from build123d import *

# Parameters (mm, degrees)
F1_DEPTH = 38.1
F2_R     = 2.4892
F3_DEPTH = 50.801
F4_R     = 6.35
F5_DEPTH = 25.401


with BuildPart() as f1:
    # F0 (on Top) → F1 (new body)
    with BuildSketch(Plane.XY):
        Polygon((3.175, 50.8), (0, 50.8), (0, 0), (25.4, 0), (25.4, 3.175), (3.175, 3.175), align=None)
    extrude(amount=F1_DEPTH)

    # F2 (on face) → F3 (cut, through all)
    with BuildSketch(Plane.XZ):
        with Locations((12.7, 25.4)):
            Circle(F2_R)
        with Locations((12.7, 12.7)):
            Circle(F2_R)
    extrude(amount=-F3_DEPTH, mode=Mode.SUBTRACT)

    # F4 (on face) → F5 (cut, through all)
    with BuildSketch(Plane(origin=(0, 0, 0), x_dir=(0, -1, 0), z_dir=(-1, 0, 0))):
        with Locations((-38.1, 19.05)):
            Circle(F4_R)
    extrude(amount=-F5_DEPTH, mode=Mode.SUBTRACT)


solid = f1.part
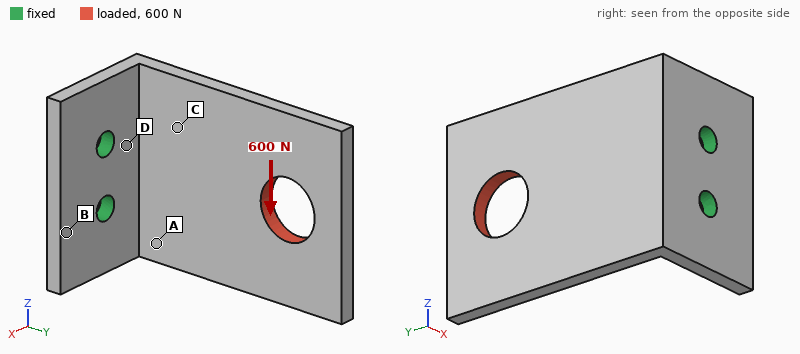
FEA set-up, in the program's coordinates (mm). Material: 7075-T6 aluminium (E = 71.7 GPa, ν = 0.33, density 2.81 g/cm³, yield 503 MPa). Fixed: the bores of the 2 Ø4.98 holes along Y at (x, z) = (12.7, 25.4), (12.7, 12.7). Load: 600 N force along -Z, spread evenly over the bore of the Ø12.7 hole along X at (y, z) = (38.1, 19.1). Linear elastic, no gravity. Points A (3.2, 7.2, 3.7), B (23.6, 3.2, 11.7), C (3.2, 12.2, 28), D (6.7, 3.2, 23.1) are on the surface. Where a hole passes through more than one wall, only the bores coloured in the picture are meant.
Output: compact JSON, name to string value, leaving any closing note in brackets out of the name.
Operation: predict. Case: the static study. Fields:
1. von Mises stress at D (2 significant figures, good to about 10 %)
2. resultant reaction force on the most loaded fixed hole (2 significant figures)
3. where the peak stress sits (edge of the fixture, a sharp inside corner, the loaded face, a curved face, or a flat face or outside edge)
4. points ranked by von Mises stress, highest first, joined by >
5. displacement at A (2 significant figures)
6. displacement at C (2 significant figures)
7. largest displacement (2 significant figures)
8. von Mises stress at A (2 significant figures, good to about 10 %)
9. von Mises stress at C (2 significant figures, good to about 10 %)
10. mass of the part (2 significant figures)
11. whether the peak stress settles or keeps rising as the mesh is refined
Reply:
{"von Mises stress at D": "130 MPa", "resultant reaction force on the most loaded fixed hole": "1.2 kN", "where the peak stress sits": "edge of the fixture", "points ranked by von Mises stress, highest first, joined by >": "D > A > C > B", "displacement at A": "0.12 mm", "displacement at C": "0.11 mm", "largest displacement": "0.42 mm", "von Mises stress at A": "83 MPa", "von Mises stress at C": "51 MPa", "mass of the part": "23 g", "whether the peak stress settles or keeps rising as the mesh is refined": "keeps rising"}
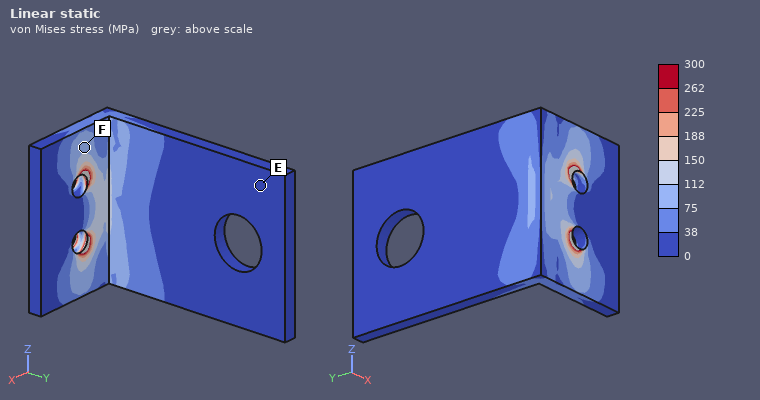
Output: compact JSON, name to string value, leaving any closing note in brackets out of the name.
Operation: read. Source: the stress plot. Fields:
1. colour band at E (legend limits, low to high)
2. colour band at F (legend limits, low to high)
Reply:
{"colour band at E": "0 to 38 MPa", "colour band at F": "75 to 112 MPa"}
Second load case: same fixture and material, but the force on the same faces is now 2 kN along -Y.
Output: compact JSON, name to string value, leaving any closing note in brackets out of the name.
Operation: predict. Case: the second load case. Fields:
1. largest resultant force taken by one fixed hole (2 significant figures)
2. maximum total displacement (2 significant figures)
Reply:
{"largest resultant force taken by one fixed hole": "1.0 kN", "maximum total displacement": "0.72 mm"}
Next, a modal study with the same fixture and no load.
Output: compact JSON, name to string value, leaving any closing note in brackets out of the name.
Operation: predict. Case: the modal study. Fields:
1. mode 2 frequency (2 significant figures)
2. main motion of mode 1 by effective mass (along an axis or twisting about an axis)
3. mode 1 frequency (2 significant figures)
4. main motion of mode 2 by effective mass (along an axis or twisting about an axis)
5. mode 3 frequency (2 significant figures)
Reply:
{"mode 2 frequency": "2200 Hz", "main motion of mode 1 by effective mass": "along X", "mode 1 frequency": "880 Hz", "main motion of mode 2 by effective mass": "along Z", "mode 3 frequency": "3000 Hz"}
